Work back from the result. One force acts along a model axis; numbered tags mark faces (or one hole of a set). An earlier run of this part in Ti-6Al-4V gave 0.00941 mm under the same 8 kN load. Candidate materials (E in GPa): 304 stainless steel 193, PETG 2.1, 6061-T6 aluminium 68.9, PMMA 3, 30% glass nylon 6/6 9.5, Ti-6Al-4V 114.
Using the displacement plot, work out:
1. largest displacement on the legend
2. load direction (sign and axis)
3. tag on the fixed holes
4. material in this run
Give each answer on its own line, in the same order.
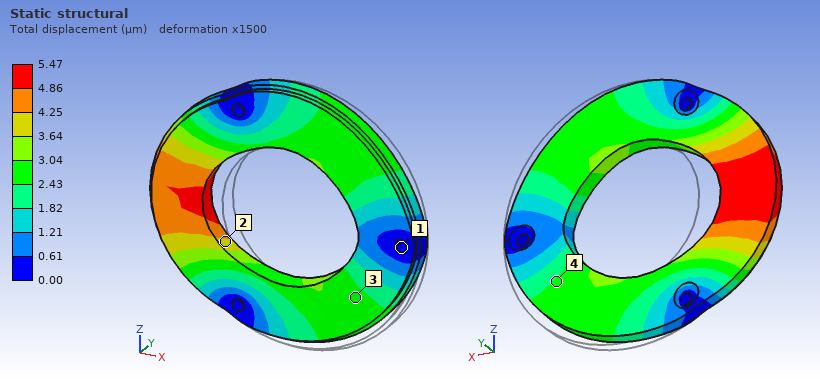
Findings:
5.47 µm
-X
1
304 stainless steel
